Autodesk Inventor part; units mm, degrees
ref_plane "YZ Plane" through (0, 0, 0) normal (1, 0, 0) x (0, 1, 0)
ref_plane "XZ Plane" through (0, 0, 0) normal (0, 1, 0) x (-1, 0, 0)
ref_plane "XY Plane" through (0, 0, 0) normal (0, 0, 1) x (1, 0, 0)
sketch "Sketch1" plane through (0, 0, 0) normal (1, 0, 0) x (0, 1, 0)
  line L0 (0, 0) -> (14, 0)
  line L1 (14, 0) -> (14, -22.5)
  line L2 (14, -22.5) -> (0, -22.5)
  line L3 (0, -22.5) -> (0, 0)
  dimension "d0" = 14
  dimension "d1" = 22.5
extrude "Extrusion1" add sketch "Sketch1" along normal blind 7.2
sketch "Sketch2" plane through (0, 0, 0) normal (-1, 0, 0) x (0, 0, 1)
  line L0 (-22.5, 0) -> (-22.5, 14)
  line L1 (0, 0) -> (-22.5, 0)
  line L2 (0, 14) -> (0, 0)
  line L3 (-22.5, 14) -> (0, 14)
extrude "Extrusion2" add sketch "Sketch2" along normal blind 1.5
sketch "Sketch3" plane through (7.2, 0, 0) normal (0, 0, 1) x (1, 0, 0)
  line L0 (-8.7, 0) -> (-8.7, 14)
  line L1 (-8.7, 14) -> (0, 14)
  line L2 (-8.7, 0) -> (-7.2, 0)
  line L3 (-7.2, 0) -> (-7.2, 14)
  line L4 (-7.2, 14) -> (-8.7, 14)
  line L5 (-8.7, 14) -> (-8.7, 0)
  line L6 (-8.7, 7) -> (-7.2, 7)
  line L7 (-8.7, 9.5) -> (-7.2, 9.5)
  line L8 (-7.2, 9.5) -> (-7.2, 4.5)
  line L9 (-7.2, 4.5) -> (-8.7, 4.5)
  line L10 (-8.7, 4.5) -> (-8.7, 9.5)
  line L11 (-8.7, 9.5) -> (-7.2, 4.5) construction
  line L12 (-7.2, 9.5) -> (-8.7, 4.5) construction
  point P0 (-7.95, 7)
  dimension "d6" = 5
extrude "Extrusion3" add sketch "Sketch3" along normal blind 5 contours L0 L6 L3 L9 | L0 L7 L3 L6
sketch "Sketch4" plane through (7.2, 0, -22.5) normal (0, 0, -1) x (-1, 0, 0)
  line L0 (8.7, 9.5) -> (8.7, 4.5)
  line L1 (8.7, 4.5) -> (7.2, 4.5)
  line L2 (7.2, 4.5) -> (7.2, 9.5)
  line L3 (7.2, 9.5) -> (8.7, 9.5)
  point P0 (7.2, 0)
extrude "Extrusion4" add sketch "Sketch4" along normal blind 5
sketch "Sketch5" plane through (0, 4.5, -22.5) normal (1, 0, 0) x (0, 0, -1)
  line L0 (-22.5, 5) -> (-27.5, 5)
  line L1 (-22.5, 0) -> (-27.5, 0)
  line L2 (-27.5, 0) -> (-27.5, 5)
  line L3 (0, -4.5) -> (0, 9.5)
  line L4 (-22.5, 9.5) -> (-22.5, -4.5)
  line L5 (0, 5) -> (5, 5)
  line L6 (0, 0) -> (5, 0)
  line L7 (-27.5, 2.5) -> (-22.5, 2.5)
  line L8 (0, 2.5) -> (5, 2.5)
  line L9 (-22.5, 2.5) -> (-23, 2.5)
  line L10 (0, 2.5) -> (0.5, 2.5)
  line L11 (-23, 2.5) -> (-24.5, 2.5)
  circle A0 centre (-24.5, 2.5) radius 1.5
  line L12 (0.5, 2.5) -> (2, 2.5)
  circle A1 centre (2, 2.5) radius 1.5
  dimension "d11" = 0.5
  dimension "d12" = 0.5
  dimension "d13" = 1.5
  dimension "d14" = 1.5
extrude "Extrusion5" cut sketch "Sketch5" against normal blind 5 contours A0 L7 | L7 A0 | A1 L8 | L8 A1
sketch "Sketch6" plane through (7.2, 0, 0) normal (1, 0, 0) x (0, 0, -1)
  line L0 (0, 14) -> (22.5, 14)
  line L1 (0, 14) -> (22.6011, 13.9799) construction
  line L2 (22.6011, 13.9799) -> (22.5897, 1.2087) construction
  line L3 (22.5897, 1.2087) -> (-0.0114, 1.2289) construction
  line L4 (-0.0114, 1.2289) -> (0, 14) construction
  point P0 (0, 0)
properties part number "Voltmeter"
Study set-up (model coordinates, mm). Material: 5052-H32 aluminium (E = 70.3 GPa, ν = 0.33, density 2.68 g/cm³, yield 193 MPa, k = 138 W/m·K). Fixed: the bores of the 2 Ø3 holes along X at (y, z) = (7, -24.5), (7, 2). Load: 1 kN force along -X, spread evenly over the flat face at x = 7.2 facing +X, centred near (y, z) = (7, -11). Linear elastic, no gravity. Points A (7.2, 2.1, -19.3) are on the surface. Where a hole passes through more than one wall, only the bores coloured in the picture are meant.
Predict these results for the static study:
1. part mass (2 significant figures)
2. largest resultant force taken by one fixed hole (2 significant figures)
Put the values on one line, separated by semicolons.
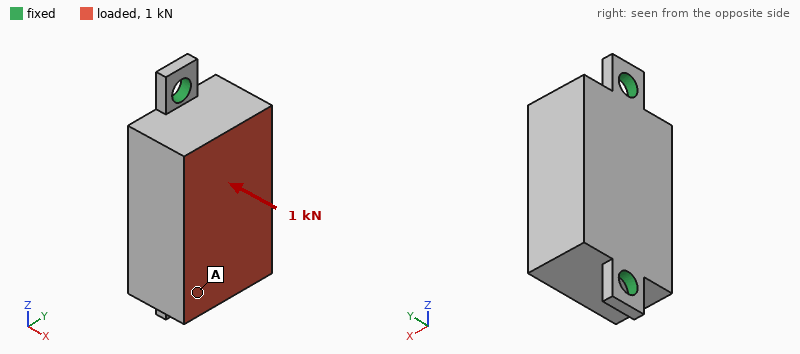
7.5 g; 580 N
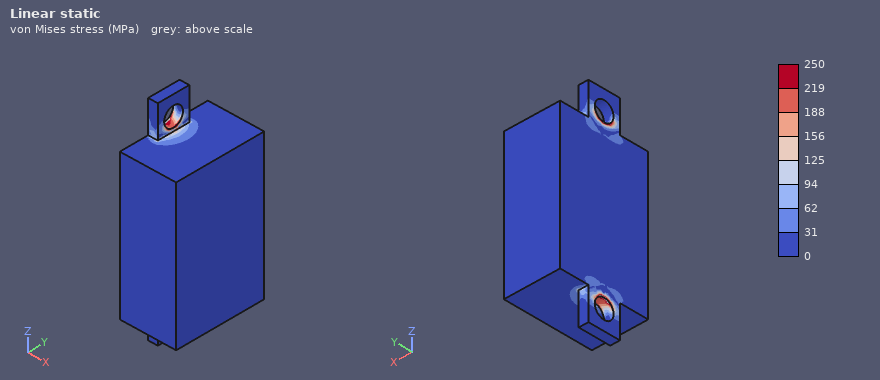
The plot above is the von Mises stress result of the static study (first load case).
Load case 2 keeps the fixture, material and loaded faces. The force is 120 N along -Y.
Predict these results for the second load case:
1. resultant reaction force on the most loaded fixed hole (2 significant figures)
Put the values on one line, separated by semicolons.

60 N
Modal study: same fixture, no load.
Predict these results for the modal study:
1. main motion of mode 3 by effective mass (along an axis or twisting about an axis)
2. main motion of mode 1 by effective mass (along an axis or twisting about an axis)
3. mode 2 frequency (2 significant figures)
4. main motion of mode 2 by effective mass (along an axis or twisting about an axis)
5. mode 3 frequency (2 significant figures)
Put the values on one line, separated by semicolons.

along Y; along Y; 20 kHz; along X; 29 kHz
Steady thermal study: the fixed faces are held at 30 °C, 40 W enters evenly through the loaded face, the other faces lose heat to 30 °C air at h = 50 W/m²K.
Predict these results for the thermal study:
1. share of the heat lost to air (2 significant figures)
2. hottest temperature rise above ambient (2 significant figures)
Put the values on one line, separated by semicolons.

5.1 %; 50 K
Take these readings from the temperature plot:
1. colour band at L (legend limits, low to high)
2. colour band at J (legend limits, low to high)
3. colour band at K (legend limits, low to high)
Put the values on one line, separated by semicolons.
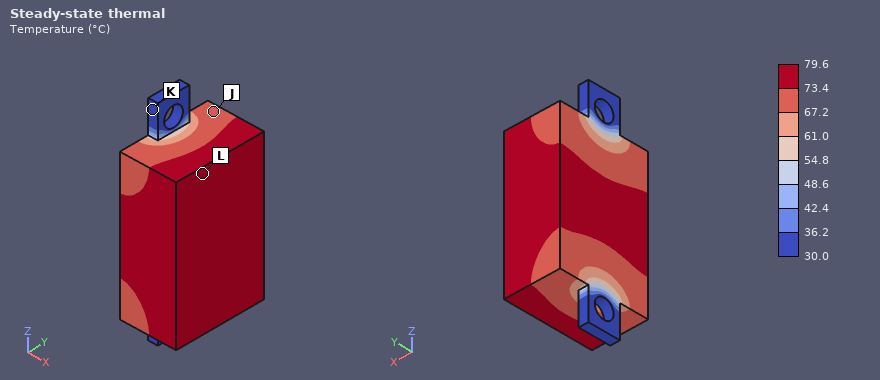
73.4 to 79.6 °C; 67.2 to 73.4 °C; 30.0 to 36.2 °C
